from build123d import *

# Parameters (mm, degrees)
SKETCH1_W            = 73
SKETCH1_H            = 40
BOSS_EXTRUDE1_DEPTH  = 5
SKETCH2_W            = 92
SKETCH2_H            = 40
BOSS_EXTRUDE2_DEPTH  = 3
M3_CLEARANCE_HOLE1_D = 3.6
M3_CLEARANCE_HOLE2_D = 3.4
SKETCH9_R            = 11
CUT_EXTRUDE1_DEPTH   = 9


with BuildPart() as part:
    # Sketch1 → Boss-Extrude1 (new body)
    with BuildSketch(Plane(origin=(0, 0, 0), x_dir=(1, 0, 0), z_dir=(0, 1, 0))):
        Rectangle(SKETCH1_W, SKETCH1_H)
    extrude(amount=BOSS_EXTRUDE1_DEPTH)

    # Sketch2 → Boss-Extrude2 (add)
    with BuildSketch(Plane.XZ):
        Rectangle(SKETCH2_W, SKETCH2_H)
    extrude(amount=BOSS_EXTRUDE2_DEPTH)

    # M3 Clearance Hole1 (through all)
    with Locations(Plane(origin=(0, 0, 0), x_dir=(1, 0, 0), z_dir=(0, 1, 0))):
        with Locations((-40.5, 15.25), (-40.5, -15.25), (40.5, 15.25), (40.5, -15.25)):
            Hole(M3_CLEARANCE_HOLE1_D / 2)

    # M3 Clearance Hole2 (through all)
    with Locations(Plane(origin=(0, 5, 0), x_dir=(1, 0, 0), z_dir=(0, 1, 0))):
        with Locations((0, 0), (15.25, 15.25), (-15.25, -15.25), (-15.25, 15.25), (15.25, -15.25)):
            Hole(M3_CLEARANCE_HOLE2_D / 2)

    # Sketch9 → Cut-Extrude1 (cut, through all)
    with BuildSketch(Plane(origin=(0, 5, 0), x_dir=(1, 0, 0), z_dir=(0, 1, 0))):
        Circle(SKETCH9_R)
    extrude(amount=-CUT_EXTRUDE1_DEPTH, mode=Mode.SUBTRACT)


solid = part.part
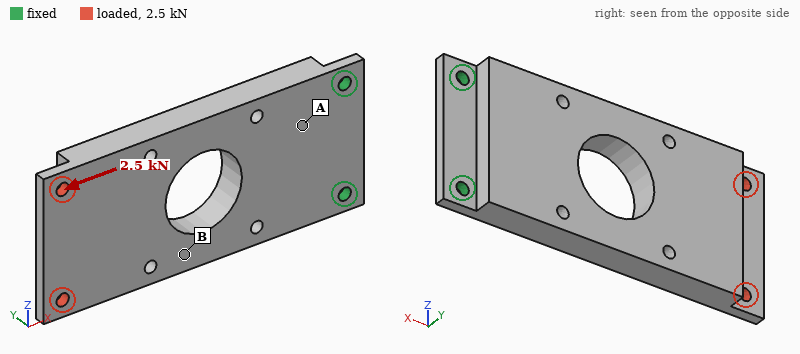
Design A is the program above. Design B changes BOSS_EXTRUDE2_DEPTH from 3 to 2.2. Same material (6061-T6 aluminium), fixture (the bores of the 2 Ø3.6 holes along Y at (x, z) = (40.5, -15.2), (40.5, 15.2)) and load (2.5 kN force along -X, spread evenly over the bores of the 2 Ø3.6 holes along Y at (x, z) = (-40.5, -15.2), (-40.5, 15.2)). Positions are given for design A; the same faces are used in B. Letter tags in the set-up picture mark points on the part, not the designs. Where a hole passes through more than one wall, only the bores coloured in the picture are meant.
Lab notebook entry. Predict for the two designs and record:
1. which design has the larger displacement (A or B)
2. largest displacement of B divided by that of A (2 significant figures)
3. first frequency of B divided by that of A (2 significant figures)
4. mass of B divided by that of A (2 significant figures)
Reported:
B
1.4
0.74
0.88
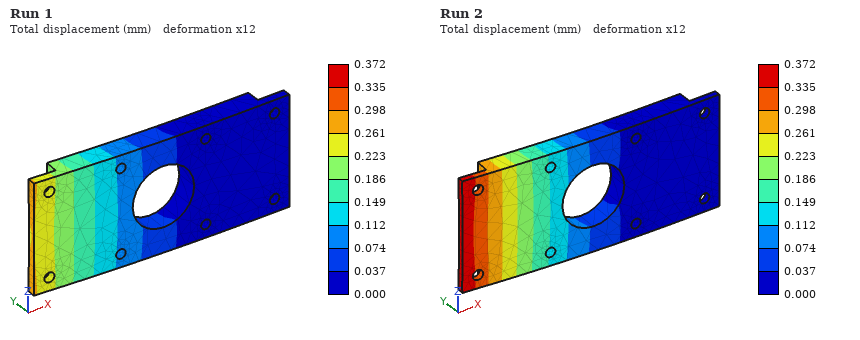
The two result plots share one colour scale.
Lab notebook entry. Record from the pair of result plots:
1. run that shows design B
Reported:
Run 2
